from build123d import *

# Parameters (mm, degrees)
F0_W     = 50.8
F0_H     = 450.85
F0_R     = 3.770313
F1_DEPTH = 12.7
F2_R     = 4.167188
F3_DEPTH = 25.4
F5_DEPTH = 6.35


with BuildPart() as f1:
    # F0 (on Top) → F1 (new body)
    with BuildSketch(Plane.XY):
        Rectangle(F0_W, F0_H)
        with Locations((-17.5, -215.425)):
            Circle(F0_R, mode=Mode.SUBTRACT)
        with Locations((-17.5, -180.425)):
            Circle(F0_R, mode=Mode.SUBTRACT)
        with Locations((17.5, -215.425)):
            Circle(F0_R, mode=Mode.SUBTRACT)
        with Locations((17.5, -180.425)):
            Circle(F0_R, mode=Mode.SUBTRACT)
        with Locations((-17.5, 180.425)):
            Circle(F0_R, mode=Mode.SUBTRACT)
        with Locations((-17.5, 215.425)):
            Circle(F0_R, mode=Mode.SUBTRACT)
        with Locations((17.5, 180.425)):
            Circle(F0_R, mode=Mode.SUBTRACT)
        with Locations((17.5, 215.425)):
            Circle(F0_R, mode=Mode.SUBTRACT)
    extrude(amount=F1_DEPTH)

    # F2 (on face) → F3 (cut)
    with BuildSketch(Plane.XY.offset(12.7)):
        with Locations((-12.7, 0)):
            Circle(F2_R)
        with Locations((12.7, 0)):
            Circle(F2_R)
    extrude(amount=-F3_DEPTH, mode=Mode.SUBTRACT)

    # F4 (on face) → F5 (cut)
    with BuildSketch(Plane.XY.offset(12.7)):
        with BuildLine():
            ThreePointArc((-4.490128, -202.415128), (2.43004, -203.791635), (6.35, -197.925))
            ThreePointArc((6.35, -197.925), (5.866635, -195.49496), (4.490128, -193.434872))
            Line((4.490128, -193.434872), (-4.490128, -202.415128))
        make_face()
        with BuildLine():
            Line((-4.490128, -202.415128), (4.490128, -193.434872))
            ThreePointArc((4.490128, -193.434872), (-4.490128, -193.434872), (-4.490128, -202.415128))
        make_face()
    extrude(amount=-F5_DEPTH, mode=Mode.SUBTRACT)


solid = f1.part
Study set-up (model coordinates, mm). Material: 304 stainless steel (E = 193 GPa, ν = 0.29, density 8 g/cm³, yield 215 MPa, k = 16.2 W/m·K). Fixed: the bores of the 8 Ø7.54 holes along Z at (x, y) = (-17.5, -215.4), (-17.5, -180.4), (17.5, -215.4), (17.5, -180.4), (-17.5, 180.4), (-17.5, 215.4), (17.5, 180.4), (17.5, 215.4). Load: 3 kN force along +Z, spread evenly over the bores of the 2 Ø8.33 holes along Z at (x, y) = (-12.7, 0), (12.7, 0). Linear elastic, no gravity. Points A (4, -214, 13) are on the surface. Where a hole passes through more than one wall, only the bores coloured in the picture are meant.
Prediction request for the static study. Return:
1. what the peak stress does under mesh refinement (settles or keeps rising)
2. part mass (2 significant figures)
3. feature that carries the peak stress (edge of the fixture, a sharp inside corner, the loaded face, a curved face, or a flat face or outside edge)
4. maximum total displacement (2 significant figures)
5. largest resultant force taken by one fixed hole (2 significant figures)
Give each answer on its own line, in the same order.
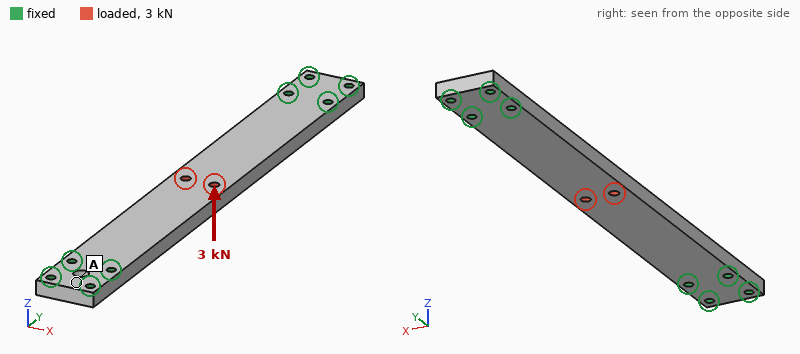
keeps rising
2.3 kg
a sharp inside corner
0.46 mm
1.2 kN
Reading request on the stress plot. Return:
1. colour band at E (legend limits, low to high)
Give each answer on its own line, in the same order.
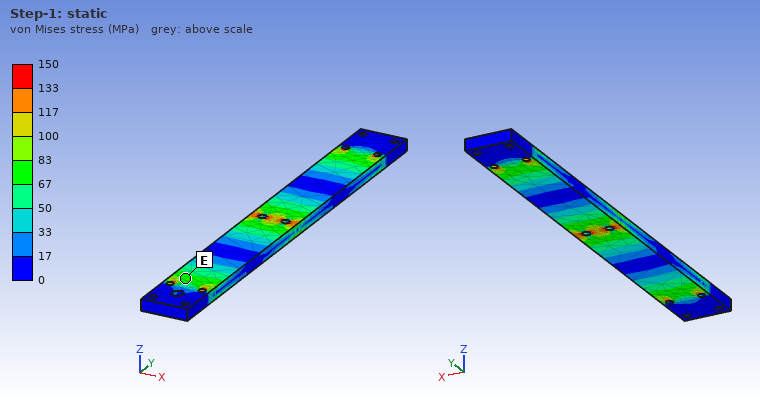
67 to 83 MPa
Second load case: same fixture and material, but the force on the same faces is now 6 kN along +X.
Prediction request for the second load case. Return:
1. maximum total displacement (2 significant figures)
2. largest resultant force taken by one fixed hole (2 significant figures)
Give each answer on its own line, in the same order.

69 µm
7.1 kN
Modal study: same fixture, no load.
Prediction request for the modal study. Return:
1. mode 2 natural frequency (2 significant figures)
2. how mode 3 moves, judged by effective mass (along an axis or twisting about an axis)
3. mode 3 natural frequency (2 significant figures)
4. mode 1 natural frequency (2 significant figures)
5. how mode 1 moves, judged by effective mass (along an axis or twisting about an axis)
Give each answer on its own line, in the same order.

1300 Hz
along X
1800 Hz
490 Hz
along Z
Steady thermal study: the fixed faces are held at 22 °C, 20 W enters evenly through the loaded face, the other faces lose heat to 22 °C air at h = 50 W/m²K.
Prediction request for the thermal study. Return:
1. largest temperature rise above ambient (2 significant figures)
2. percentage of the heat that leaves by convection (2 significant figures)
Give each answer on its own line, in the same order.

41 K
98 %
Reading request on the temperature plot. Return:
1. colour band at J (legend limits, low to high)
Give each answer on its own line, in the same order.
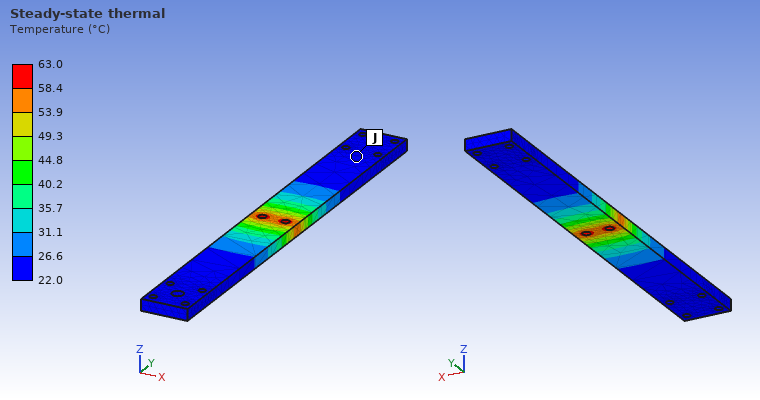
22.0 to 26.6 °C
